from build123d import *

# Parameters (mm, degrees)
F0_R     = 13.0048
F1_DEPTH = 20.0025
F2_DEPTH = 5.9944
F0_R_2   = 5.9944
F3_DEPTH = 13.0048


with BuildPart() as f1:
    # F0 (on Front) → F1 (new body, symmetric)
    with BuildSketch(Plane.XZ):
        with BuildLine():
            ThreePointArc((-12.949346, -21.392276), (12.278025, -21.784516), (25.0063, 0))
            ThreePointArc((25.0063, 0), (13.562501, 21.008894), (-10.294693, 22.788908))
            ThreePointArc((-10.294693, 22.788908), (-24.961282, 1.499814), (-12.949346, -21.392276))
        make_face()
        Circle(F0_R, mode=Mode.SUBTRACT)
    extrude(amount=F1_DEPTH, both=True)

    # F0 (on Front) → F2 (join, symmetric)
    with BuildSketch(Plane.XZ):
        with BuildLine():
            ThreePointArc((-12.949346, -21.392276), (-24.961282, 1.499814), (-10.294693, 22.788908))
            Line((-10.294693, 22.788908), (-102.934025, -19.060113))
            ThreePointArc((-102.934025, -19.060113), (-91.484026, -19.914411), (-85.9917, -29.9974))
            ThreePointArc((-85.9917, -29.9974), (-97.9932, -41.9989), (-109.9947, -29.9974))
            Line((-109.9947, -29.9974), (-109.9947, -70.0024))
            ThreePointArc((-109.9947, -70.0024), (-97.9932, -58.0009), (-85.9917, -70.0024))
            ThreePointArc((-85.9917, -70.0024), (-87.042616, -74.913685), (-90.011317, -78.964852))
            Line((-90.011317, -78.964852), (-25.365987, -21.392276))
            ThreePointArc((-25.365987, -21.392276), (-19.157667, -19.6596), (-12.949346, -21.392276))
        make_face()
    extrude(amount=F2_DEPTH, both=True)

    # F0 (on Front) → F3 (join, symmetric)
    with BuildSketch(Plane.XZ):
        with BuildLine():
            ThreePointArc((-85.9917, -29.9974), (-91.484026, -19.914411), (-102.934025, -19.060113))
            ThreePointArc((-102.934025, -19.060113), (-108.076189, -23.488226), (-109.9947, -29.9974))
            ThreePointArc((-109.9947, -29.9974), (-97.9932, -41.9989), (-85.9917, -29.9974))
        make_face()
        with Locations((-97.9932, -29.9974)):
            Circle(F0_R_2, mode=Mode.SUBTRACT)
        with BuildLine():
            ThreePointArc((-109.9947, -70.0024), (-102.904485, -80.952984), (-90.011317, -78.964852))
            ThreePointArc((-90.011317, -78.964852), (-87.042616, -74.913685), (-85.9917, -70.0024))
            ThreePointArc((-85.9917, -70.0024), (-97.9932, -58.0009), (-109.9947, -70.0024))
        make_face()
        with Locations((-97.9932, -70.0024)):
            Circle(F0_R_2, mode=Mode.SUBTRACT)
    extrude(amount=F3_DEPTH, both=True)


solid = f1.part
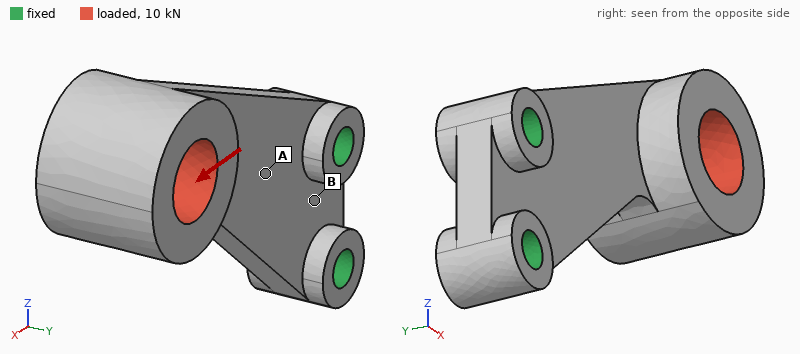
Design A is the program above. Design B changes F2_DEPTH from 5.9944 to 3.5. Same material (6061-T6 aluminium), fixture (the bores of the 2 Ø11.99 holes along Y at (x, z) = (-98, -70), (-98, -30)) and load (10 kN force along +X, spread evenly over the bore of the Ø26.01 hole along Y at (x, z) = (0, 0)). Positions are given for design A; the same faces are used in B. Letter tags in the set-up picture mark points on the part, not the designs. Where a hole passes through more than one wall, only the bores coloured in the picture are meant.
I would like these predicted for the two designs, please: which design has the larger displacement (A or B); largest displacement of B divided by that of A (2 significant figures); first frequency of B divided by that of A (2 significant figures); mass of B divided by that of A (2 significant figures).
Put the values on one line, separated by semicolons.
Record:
B; 1.7; 0.47; 0.84
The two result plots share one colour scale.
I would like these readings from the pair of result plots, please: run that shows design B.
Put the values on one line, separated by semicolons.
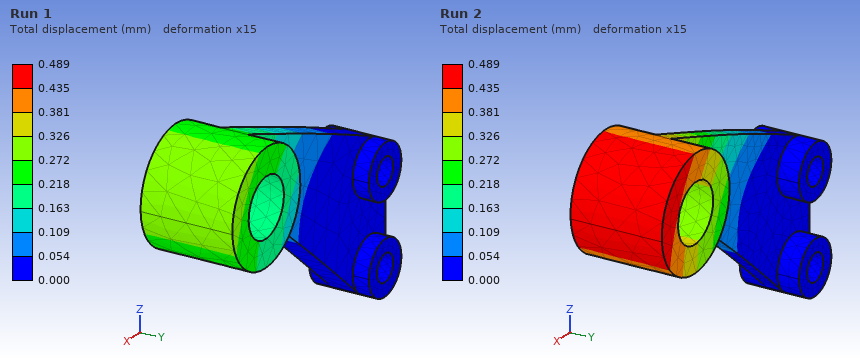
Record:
Run 2
